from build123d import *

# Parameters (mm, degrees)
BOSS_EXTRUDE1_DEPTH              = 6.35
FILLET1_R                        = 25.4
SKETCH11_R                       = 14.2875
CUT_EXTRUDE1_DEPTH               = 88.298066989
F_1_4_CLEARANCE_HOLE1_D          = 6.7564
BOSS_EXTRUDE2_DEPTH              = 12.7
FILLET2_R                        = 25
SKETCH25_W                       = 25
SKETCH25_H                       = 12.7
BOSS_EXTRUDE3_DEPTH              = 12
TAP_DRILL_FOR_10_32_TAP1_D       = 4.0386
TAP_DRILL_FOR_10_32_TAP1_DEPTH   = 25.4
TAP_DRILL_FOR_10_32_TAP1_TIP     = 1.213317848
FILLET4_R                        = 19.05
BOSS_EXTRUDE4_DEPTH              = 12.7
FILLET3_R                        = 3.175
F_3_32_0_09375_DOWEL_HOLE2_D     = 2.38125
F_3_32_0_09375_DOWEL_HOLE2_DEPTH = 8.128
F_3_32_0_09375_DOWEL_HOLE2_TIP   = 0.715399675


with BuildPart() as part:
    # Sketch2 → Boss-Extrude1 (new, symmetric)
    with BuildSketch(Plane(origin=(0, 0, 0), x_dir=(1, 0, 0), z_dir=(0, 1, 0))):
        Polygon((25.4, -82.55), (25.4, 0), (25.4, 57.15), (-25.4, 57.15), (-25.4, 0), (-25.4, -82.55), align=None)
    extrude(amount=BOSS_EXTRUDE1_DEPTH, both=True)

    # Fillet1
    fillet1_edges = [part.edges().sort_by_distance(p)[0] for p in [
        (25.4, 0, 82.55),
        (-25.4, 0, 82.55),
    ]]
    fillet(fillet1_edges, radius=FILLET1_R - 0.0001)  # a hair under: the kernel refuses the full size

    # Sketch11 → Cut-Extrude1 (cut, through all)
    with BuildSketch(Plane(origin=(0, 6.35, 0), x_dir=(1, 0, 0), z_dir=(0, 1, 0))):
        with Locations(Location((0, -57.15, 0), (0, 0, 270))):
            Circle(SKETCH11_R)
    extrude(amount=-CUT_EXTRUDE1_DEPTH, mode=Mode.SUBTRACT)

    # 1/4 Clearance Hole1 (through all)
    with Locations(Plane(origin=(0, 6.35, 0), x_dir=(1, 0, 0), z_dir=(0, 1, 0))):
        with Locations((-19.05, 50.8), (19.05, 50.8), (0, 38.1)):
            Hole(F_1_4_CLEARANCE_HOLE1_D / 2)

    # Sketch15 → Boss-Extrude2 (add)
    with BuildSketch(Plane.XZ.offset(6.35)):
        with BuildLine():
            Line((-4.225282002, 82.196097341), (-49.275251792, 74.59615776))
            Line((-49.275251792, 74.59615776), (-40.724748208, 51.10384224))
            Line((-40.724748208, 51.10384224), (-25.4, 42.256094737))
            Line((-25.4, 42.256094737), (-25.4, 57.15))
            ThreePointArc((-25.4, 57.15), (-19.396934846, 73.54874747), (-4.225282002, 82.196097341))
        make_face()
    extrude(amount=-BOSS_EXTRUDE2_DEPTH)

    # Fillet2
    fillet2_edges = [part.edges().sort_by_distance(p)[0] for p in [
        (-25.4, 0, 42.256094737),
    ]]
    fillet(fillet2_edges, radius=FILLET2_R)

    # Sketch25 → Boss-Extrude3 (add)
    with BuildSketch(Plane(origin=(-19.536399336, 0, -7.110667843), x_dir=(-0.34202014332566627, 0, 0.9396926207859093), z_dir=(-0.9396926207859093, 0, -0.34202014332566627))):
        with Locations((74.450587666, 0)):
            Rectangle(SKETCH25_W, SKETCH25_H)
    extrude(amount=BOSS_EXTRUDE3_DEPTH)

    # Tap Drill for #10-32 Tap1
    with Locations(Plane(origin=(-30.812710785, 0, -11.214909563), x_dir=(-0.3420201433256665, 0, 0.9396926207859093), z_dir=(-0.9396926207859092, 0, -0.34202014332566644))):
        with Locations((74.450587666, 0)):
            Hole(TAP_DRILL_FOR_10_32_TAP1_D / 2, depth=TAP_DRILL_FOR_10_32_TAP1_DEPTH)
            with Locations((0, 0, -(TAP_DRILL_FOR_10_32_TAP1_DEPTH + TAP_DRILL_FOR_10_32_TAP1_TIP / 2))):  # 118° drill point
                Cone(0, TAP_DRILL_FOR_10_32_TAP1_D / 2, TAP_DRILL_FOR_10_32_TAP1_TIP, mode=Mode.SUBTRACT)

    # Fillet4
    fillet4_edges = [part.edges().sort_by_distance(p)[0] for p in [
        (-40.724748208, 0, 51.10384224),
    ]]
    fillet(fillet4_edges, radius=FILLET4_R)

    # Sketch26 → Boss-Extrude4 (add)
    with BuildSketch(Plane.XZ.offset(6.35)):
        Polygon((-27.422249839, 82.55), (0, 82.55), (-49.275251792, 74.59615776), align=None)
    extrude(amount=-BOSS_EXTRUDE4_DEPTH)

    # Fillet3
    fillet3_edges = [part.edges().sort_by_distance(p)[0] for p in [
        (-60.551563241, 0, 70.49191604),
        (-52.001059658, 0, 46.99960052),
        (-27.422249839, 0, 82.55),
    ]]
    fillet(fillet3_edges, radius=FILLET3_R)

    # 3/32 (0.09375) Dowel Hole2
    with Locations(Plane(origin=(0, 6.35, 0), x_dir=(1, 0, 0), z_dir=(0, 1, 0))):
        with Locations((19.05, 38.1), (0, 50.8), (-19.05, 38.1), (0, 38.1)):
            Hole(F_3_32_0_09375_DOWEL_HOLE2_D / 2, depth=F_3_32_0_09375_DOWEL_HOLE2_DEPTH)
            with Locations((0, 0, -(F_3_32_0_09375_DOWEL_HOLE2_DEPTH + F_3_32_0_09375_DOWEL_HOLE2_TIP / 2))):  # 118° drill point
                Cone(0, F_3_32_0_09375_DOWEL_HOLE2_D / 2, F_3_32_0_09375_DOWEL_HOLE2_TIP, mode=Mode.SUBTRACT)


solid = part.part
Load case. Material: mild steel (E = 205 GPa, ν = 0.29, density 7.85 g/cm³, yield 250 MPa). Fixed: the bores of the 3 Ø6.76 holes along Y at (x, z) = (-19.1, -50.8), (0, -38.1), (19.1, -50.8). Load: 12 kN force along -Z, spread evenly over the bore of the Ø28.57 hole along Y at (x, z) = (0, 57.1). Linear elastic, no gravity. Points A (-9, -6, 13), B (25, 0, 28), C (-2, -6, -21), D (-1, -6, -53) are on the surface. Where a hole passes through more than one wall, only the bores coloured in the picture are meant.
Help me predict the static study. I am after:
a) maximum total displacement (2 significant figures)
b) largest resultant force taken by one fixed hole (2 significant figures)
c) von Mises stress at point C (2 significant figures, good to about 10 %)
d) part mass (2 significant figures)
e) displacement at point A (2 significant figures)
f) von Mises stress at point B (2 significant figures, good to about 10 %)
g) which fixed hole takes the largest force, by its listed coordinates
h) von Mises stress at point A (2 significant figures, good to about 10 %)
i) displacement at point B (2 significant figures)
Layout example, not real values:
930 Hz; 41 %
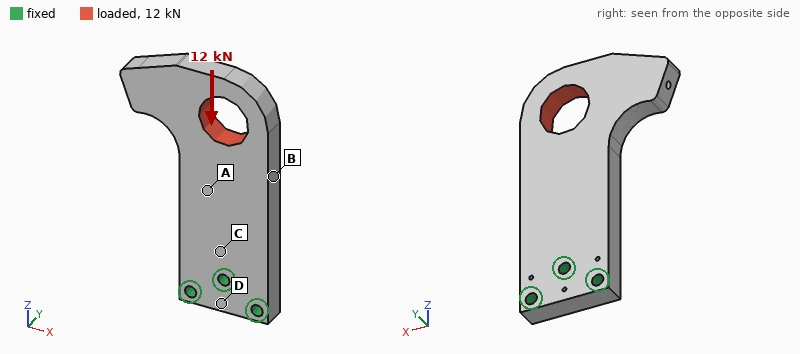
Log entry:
15 µm; 6.2 kN; 23 MPa; 710 g; 5.1 µm; 27 MPa; (0, -38.1); 17 MPa; 7.1 µm
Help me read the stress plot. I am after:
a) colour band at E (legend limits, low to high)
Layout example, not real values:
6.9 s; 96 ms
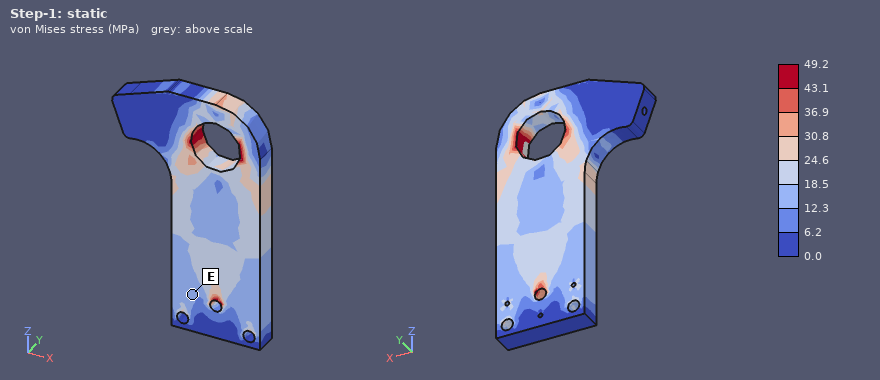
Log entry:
12.3 to 18.5 MPa
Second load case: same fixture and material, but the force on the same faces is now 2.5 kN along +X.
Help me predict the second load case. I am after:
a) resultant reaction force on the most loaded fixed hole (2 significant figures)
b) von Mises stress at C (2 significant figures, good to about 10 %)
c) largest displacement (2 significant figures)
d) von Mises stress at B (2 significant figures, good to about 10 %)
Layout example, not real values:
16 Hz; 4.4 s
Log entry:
5.5 kN; 9.9 MPa; 61 µm; 16 MPa
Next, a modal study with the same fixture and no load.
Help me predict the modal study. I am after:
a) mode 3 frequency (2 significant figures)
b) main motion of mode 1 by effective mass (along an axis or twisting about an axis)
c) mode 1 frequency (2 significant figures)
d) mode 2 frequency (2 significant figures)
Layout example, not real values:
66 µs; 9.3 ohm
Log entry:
2000 Hz; along Y; 650 Hz; 2000 Hz
